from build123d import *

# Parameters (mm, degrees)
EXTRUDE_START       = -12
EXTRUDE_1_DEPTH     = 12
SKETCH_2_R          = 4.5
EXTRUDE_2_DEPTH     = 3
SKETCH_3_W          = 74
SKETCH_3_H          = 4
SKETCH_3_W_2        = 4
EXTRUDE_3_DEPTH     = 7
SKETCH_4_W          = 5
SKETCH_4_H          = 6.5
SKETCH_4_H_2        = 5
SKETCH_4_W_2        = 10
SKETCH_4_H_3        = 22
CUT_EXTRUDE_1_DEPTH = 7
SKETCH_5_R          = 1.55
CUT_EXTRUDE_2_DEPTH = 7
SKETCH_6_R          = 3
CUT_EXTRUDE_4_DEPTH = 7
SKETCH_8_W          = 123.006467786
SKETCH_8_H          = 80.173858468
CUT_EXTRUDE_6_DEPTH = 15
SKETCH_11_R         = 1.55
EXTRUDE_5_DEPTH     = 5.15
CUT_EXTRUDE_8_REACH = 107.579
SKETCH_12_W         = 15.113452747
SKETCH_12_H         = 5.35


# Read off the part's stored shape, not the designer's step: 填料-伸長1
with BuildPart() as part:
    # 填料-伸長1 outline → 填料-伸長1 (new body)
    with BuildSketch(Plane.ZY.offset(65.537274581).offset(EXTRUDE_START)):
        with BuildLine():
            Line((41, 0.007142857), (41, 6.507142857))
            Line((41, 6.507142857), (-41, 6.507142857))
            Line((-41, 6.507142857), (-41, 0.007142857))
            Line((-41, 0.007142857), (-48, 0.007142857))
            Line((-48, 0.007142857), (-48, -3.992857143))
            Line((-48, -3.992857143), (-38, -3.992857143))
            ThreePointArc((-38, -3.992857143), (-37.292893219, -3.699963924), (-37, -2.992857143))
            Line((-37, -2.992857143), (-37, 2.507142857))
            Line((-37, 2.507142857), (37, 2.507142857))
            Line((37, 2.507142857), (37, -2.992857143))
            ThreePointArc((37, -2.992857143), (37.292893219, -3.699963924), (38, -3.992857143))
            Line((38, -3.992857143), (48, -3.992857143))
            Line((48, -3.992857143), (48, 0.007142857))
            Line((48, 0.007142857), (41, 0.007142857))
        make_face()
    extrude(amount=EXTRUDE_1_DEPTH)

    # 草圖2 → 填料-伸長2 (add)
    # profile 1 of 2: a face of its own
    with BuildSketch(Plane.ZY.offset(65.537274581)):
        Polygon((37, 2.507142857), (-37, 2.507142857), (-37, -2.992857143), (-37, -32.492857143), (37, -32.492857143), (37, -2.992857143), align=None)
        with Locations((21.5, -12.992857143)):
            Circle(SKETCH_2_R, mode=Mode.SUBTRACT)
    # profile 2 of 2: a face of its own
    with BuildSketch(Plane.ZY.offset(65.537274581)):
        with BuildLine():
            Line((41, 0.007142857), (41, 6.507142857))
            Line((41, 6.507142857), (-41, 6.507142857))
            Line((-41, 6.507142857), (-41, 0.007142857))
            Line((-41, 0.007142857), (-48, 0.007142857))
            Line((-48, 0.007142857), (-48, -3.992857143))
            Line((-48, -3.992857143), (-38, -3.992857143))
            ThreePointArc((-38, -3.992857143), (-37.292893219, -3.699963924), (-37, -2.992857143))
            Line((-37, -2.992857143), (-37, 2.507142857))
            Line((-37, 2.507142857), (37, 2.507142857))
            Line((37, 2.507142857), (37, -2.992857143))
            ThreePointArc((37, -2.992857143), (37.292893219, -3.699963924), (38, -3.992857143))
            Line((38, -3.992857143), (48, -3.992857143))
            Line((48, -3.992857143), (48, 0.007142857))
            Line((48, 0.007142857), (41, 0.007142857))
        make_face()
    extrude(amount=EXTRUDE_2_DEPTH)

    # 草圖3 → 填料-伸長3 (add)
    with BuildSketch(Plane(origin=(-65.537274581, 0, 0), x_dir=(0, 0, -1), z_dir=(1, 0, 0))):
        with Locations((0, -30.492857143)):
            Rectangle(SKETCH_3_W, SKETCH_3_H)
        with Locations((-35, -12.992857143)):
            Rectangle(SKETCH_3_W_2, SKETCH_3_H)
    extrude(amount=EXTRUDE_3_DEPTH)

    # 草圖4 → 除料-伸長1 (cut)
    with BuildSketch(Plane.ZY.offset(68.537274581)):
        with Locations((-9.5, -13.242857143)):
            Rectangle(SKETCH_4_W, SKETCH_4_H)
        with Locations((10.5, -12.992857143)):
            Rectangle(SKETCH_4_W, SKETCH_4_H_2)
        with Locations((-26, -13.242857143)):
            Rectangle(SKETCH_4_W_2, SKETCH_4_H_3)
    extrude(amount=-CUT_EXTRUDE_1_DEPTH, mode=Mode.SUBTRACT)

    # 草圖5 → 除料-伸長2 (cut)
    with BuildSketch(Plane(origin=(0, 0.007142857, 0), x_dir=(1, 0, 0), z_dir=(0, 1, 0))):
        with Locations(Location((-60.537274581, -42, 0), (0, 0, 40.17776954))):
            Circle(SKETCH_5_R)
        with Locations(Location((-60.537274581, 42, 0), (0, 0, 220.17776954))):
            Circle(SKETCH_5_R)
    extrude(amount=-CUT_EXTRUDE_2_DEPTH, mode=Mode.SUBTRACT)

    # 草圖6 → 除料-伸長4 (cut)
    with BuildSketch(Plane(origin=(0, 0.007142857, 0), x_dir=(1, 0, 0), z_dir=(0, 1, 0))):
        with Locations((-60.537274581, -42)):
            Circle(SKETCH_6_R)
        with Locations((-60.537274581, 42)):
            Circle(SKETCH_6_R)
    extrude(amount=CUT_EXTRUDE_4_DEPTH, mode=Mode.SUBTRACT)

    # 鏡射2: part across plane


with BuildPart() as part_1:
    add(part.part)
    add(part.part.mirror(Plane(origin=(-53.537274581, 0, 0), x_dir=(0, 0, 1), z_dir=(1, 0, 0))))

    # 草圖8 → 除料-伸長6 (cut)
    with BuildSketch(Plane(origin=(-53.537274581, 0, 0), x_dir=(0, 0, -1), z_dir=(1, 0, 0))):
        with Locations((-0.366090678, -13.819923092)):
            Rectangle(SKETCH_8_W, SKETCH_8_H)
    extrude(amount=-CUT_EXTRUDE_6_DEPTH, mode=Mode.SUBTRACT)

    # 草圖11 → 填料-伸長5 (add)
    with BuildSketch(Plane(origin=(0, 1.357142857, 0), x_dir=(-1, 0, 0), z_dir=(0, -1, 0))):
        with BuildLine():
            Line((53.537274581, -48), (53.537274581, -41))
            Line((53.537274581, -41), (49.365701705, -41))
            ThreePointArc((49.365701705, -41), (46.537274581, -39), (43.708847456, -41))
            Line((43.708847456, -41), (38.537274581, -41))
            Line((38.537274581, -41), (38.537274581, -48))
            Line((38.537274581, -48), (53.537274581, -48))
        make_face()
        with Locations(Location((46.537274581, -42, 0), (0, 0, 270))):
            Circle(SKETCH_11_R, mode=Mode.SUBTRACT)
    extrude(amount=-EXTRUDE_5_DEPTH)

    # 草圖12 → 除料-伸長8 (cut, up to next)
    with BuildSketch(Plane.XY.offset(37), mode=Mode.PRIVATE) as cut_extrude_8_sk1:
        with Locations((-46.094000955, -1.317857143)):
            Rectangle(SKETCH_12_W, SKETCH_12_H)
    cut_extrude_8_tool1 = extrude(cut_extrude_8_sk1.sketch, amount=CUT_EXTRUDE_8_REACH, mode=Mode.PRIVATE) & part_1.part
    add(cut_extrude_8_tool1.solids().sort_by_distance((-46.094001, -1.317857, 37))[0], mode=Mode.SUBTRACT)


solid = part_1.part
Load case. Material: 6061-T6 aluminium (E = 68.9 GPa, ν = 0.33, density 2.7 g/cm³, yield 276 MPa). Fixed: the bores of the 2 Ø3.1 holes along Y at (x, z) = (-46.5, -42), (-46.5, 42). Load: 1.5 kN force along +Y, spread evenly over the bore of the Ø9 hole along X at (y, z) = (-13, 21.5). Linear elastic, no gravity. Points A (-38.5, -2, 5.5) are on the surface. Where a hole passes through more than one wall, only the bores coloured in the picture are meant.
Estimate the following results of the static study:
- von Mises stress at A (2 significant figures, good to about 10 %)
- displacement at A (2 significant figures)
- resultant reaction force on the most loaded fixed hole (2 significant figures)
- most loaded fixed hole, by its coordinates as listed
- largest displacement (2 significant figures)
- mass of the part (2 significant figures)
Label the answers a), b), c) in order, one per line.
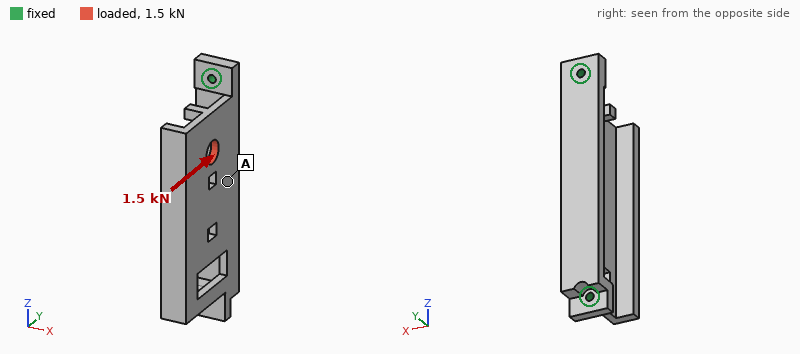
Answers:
a) 13 MPa
b) 0.062 mm
c) 1.2 kN
d) (-46.5, 42)
e) 0.16 mm
f) 41 g
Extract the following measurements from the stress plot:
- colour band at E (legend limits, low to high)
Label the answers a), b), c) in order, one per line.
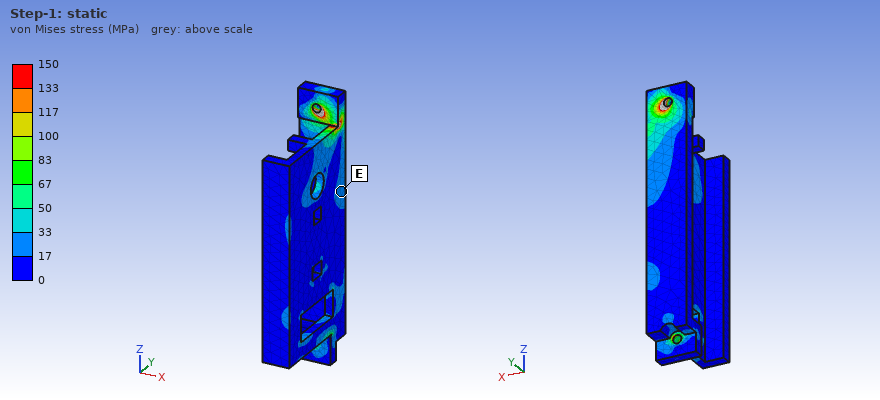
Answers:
a) 17 to 33 MPa
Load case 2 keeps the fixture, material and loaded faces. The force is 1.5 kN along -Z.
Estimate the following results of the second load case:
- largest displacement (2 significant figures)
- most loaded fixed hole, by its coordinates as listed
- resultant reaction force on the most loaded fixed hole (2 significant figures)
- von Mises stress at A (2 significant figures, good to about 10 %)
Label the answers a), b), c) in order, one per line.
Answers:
a) 50 µm
b) (-46.5, 42)
c) 1.2 kN
d) 11 MPa
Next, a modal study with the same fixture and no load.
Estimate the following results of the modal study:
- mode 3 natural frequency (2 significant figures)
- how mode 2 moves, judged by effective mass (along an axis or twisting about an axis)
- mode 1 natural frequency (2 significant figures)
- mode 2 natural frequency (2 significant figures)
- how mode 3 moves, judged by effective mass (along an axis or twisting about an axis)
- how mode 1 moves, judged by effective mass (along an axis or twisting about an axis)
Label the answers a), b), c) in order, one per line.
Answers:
a) 4300 Hz
b) twisting about Y
c) 960 Hz
d) 2100 Hz
e) along Y
f) along X
